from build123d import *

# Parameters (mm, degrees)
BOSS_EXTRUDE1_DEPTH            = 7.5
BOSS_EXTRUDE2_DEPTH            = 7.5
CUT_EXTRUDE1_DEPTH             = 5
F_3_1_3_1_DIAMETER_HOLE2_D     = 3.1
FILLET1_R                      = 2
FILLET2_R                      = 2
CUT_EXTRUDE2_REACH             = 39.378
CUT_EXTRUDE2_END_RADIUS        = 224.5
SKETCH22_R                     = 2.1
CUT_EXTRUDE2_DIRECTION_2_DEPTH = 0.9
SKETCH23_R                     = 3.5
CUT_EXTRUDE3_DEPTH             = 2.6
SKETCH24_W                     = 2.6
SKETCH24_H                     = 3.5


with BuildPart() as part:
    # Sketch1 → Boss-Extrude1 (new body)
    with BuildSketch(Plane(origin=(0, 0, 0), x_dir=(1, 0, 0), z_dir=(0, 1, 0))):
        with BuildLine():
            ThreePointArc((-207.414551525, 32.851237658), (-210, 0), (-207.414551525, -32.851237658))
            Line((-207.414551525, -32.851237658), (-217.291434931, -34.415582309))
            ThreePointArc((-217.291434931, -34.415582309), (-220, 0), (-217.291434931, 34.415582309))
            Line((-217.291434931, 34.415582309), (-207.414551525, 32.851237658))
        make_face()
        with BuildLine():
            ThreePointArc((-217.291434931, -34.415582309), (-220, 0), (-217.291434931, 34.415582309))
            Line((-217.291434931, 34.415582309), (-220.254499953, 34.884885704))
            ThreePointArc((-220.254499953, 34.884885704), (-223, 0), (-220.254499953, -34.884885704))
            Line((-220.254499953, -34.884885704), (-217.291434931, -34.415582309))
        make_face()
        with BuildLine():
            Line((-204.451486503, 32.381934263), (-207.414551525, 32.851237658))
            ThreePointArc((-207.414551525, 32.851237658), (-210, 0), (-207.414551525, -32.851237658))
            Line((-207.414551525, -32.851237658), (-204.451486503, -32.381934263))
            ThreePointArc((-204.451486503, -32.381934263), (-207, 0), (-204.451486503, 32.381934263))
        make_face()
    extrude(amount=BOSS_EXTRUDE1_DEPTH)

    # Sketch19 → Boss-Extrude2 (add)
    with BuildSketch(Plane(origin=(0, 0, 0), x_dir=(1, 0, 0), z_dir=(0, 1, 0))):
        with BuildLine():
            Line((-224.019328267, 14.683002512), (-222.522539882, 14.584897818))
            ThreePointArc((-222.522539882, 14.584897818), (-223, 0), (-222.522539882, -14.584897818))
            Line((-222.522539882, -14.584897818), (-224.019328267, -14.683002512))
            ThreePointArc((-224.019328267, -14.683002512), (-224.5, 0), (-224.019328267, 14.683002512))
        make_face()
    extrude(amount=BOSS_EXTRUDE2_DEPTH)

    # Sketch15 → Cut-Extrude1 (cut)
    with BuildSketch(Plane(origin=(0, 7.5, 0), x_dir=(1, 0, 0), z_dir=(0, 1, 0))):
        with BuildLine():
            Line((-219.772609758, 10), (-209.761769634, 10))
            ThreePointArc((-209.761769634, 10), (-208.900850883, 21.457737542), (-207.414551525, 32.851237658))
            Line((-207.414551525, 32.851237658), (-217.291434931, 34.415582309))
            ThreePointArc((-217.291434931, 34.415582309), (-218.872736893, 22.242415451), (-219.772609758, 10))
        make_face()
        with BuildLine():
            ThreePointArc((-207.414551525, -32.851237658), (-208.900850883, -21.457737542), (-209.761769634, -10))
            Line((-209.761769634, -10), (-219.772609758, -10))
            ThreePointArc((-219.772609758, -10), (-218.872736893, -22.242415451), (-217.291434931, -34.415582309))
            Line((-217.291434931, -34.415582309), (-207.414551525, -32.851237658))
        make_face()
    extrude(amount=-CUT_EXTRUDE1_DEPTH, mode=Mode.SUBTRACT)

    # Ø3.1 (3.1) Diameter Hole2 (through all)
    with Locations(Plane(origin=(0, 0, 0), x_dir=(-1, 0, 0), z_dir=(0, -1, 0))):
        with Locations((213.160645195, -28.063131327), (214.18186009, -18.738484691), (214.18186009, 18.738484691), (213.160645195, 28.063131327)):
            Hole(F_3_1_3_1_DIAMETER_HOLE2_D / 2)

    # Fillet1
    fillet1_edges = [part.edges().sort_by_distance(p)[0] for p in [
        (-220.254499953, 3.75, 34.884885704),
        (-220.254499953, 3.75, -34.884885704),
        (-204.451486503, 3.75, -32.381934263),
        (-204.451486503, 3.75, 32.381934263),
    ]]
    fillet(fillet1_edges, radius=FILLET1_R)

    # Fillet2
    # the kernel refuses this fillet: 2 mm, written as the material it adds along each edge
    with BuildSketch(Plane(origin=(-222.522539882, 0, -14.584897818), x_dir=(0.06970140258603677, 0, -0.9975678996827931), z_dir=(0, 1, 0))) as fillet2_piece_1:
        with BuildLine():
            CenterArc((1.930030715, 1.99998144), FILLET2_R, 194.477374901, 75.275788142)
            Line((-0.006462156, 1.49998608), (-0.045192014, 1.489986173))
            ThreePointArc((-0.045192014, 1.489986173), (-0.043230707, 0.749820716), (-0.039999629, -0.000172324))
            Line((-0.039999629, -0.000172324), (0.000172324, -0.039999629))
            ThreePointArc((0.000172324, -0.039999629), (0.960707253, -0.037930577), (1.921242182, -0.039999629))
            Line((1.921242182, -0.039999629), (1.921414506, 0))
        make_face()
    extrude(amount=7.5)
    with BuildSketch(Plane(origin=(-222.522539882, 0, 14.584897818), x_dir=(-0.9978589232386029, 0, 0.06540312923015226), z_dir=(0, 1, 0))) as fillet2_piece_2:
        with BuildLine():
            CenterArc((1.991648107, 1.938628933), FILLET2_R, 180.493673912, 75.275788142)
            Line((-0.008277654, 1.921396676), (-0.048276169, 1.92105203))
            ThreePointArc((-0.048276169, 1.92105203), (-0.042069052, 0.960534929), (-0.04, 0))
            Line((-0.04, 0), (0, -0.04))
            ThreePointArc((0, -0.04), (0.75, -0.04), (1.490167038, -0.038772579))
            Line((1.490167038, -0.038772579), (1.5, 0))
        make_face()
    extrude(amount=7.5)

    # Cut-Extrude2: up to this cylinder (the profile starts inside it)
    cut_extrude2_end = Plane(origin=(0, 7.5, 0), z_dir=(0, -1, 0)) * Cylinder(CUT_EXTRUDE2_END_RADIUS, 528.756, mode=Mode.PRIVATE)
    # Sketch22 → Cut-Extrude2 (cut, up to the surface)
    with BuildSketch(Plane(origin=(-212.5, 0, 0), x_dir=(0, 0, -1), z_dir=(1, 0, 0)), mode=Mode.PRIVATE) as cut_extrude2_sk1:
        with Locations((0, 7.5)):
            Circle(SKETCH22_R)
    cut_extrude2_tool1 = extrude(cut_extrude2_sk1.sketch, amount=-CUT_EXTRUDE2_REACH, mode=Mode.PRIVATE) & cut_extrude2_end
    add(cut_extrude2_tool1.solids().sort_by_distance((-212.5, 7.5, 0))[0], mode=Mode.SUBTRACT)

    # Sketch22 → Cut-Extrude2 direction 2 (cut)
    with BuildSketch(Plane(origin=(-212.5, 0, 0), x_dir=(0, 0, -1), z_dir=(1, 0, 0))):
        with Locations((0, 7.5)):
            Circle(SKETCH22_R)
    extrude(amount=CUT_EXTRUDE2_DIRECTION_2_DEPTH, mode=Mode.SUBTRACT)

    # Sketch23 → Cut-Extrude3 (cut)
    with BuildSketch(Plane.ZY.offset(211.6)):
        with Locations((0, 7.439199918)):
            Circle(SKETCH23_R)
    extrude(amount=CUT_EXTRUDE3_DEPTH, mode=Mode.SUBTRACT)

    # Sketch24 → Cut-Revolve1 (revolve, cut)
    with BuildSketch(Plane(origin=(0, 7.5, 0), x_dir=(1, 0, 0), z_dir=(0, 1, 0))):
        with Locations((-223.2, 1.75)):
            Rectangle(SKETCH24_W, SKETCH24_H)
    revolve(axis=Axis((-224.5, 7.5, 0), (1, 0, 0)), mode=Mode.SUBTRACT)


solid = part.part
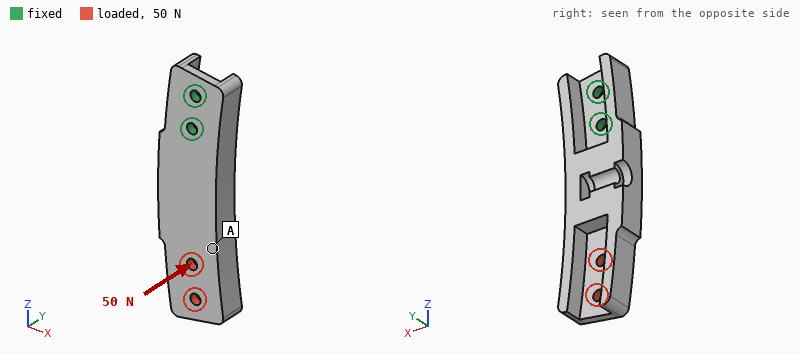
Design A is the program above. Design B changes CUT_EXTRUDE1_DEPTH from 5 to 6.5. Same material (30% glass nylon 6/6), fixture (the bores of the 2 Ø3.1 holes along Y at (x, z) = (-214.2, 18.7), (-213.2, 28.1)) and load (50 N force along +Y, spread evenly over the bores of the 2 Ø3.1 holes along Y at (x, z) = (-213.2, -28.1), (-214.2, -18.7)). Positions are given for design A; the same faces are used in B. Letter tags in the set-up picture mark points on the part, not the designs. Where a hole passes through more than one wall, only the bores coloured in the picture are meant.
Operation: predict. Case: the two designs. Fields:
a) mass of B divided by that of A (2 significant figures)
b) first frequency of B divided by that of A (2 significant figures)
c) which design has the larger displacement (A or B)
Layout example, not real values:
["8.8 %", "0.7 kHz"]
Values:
["0.89", "0.62", "B"]
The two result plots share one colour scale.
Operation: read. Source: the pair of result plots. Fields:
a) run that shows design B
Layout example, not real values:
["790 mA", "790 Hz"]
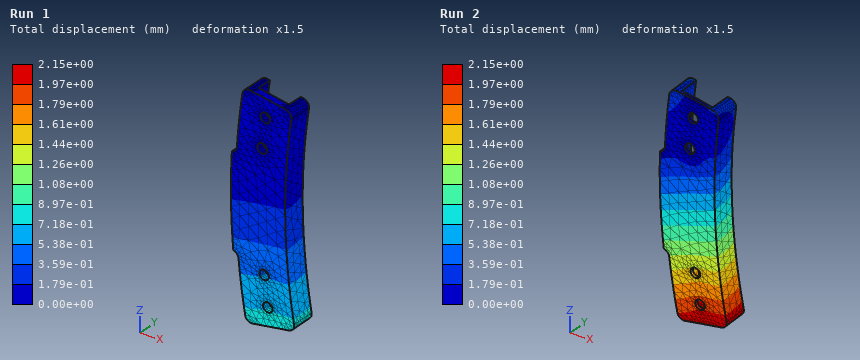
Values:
["Run 2"]
